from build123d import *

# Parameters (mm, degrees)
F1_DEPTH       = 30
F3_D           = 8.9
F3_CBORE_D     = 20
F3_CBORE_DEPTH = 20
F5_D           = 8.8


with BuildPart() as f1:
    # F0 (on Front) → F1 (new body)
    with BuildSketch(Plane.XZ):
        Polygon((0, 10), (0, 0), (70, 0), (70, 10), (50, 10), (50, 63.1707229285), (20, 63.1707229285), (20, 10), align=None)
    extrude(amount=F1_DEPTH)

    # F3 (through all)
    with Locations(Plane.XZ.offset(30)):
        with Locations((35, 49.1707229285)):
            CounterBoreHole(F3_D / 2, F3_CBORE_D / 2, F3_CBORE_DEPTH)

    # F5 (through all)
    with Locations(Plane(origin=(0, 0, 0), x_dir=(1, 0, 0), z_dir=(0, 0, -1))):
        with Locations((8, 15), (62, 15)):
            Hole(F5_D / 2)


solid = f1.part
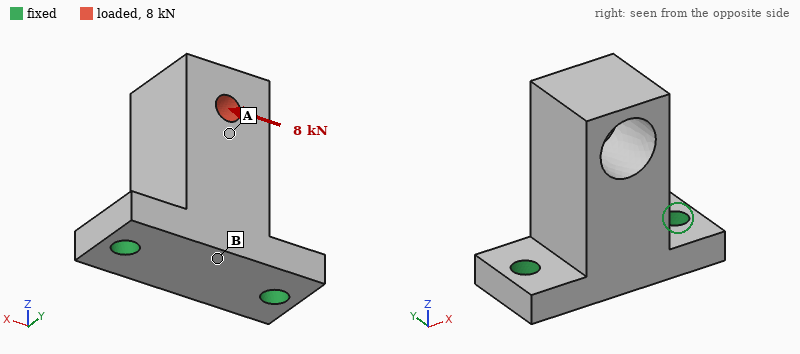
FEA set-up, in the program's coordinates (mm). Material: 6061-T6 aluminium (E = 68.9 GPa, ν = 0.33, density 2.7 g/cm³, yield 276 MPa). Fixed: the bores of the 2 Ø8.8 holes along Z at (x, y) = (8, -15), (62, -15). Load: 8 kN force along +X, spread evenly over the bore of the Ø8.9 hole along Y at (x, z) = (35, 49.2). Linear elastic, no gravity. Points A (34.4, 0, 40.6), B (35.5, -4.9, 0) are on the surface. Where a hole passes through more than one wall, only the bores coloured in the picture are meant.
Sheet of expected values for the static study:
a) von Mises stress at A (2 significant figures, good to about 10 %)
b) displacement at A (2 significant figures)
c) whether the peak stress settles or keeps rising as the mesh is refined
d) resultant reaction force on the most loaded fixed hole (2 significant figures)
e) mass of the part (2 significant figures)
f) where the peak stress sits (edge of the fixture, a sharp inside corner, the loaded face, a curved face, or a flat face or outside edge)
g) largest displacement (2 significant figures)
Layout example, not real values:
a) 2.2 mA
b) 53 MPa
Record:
a) 67 MPa
b) 0.11 mm
c) keeps rising
d) 9.6 kN
e) 160 g
f) edge of the fixture
g) 0.21 mm
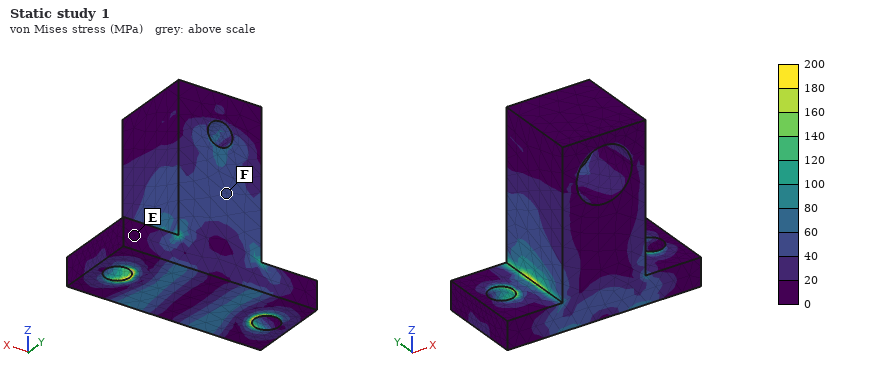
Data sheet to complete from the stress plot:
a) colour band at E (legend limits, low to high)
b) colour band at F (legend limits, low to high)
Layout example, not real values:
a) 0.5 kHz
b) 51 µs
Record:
a) 0 to 20 MPa
b) 40 to 60 MPa
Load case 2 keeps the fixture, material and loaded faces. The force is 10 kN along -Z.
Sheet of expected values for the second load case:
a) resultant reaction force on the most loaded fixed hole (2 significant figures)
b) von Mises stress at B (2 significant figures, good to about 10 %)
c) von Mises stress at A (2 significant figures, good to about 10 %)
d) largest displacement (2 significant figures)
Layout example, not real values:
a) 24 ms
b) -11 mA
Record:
a) 5.3 kN
b) 37 MPa
c) 42 MPa
d) 0.20 mm
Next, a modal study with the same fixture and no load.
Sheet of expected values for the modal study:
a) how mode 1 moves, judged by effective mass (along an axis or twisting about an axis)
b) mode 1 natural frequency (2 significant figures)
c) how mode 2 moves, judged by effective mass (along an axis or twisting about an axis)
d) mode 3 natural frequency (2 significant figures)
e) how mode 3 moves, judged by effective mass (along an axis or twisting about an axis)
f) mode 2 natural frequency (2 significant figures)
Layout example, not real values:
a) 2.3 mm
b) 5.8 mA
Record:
a) along Y
b) 2500 Hz
c) along X
d) 8900 Hz
e) along Z
f) 4800 Hz
